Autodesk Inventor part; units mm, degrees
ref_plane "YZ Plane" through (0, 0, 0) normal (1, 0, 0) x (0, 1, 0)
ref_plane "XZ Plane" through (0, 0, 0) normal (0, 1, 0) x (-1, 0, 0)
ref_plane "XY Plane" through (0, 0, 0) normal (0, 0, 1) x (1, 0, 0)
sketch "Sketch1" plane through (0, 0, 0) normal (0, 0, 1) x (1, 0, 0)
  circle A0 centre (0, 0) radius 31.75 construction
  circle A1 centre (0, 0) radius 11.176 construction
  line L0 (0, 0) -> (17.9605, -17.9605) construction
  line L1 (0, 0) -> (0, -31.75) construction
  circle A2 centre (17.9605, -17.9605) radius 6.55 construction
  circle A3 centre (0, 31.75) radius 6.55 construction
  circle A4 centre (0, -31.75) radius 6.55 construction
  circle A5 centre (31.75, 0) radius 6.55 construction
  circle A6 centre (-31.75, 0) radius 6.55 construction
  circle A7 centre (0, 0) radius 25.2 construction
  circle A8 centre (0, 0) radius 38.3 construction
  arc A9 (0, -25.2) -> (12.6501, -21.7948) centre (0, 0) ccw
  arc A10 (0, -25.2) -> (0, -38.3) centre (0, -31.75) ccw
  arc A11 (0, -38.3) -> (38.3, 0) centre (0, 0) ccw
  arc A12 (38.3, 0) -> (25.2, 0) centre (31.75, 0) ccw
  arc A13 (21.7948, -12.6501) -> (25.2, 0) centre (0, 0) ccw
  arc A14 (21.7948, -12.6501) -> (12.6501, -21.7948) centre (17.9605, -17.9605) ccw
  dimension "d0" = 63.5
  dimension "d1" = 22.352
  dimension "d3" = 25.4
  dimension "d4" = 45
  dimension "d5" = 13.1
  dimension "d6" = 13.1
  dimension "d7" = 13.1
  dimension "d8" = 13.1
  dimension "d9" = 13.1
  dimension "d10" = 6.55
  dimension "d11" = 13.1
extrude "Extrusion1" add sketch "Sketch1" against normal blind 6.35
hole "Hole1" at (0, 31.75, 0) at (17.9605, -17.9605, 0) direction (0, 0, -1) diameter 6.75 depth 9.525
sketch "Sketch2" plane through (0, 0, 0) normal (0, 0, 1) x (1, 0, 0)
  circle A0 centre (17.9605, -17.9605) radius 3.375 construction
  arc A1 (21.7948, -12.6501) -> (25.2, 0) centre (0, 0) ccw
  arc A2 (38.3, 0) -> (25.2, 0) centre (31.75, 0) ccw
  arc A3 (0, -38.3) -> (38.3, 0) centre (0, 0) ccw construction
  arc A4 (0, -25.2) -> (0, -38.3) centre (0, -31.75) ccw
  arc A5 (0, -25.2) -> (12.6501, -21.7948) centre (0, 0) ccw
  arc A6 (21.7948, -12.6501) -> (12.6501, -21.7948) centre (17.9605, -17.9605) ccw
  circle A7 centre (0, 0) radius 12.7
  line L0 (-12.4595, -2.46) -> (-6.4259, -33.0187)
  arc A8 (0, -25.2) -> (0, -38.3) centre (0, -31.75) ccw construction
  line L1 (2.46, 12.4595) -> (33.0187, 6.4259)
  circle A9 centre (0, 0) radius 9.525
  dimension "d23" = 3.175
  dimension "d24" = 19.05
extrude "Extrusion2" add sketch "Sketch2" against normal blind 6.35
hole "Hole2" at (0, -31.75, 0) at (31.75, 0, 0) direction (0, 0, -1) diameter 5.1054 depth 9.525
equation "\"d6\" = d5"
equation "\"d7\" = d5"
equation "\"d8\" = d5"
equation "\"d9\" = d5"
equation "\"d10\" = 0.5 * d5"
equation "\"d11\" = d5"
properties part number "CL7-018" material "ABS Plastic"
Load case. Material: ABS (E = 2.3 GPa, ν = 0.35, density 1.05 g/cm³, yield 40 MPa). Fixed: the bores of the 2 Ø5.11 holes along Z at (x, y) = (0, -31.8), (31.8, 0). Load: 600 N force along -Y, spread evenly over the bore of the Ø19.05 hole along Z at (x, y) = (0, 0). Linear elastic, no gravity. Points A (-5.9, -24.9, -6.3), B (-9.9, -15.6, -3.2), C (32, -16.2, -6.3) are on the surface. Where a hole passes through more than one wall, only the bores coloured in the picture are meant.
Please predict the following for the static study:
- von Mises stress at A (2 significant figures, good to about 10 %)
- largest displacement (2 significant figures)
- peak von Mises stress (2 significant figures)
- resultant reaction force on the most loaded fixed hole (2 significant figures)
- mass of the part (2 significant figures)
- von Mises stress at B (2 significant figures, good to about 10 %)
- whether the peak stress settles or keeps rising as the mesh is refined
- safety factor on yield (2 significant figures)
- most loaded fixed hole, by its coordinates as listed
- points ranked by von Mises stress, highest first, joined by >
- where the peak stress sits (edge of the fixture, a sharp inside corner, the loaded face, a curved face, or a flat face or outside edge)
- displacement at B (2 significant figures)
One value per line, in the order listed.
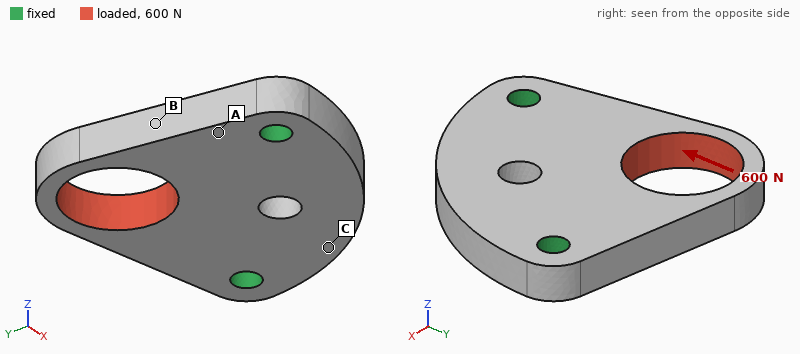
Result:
6.3 MPa
0.29 mm
24 MPa
490 N
11 g
12 MPa
settles
1.7
(0, -31.8)
B > A > C
the loaded face
0.065 mm
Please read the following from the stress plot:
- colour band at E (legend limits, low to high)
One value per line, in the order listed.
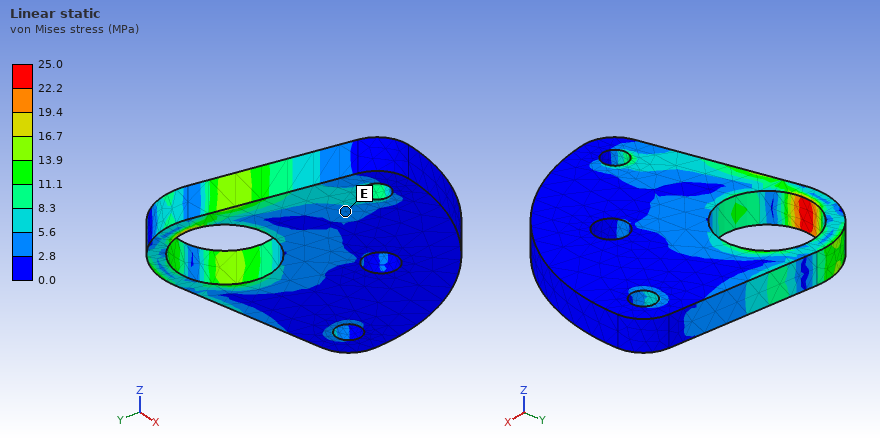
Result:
2.8 to 5.6 MPa
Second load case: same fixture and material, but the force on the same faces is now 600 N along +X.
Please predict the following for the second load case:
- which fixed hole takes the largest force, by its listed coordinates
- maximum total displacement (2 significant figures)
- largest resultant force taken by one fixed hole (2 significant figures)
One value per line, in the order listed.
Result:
(31.8, 0)
0.29 mm
490 N
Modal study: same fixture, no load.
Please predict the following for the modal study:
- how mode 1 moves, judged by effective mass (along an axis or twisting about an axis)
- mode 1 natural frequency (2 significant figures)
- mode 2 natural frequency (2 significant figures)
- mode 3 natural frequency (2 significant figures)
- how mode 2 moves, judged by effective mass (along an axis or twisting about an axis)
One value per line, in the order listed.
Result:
along Z
1700 Hz
3600 Hz
4000 Hz
along Z
